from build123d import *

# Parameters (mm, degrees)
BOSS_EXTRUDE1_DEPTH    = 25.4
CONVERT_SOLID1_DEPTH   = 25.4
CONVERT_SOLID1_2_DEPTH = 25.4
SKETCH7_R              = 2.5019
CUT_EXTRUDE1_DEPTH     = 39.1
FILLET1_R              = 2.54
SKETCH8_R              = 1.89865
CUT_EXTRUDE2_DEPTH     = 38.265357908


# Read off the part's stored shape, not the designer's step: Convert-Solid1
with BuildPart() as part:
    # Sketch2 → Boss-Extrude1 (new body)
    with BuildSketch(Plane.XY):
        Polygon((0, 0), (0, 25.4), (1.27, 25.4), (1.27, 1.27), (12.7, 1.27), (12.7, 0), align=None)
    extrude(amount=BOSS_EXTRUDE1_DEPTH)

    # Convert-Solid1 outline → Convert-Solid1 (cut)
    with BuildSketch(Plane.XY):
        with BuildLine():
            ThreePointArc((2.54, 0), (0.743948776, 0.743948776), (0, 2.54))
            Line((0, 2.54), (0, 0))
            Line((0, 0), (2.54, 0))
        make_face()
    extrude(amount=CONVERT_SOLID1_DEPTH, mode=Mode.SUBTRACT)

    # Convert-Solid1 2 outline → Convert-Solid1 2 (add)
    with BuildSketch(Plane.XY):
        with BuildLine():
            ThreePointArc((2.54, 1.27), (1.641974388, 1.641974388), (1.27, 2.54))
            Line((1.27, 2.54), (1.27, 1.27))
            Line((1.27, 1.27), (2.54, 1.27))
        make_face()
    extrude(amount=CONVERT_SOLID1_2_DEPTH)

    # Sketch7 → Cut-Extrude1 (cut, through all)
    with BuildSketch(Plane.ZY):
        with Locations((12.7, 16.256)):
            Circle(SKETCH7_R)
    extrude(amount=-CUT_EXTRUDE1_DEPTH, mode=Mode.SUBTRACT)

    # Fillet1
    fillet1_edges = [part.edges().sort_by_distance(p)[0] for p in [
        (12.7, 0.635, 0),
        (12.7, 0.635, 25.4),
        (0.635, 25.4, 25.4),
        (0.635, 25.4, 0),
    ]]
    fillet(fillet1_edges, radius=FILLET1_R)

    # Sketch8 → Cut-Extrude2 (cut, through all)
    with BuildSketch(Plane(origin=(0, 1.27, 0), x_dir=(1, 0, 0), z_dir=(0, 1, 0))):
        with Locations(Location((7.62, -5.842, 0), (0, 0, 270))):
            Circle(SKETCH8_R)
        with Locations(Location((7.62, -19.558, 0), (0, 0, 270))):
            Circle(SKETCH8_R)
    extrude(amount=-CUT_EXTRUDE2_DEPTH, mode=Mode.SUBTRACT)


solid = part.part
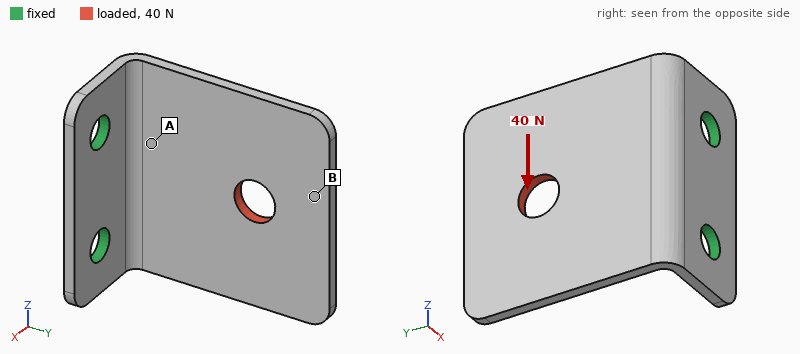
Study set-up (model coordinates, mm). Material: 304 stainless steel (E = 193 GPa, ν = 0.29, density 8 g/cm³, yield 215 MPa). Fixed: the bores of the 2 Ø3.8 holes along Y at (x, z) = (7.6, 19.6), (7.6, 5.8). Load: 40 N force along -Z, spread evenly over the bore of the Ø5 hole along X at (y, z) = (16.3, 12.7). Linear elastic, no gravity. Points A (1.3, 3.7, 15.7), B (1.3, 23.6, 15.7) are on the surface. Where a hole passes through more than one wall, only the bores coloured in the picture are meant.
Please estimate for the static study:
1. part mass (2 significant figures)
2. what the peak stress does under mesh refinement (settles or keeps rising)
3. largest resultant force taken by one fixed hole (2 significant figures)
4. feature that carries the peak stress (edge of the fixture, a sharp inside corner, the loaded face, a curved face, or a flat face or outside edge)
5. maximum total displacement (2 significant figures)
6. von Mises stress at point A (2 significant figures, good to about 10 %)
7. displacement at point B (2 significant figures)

8.8 g
keeps rising
46 N
edge of the fixture
18 µm
16 MPa
14 µm
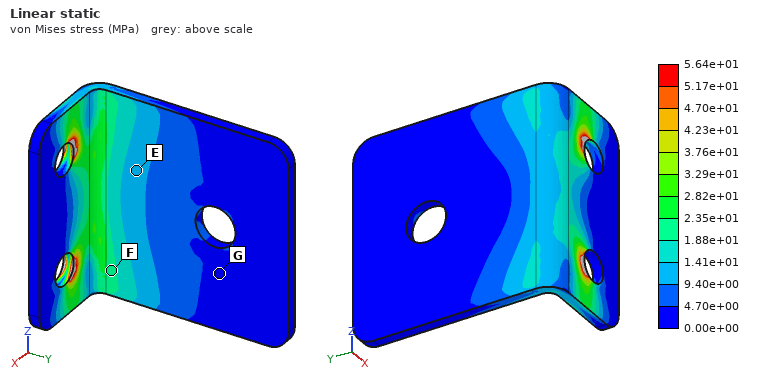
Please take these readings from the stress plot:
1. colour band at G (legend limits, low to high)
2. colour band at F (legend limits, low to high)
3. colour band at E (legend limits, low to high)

0.00e+00 to 4.70e+00 MPa
1.88e+01 to 2.35e+01 MPa
9.40e+00 to 1.41e+01 MPa
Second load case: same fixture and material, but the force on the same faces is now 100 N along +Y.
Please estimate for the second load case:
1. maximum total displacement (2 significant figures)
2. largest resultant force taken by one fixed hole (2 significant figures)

52 µm
50 N
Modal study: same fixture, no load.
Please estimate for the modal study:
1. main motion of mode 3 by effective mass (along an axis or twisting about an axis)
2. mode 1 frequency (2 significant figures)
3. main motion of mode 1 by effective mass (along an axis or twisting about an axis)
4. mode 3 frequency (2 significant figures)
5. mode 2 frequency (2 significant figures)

along Z
1300 Hz
along X
4900 Hz
3200 Hz
